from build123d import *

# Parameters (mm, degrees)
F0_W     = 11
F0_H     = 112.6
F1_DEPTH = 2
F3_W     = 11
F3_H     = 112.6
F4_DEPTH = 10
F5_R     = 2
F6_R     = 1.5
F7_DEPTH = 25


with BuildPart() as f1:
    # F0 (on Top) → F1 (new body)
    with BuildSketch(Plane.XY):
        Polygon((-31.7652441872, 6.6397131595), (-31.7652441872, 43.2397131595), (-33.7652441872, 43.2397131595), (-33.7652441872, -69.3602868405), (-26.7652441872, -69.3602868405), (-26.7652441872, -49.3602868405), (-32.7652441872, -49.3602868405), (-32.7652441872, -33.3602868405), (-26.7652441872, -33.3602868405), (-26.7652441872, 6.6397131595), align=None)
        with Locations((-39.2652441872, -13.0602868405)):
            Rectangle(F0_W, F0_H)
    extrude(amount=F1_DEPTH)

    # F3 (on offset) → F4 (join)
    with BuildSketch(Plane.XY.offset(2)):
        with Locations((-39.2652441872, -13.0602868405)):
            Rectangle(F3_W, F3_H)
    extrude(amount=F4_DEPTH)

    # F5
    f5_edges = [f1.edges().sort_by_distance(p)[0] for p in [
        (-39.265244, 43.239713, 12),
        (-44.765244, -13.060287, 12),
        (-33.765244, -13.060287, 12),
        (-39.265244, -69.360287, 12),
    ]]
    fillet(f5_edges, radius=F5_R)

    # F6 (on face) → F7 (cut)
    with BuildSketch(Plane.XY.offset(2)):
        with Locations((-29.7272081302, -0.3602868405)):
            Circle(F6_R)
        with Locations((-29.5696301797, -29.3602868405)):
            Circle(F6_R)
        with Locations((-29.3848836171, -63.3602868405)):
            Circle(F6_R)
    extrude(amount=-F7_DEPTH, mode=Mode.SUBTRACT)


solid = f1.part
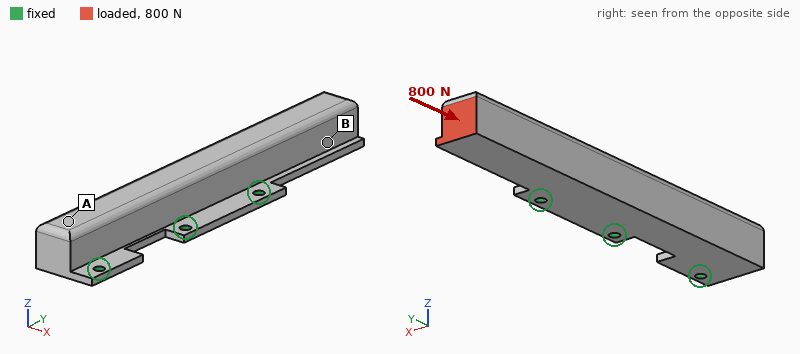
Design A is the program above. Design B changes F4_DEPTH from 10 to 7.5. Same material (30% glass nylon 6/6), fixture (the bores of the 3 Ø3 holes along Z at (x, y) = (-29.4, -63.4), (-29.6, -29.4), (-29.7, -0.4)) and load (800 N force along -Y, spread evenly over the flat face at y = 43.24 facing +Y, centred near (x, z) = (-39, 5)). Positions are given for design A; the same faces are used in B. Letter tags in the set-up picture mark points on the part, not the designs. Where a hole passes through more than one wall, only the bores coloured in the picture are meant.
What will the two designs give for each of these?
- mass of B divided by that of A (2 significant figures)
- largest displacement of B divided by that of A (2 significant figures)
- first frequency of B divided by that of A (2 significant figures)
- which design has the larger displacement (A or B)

0.80
1.5
1.1
B
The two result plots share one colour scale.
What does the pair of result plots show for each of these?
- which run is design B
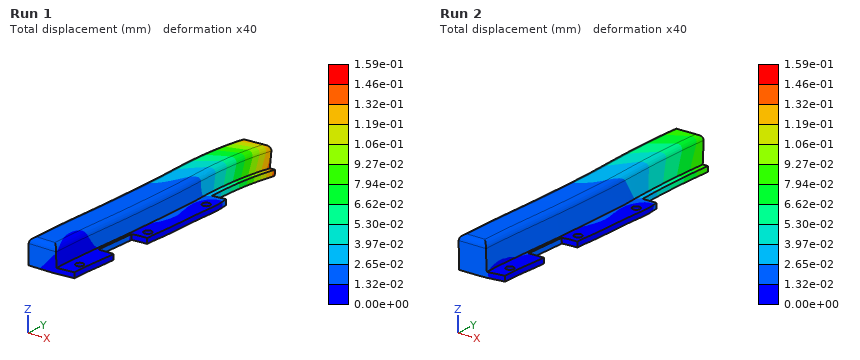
Run 1
